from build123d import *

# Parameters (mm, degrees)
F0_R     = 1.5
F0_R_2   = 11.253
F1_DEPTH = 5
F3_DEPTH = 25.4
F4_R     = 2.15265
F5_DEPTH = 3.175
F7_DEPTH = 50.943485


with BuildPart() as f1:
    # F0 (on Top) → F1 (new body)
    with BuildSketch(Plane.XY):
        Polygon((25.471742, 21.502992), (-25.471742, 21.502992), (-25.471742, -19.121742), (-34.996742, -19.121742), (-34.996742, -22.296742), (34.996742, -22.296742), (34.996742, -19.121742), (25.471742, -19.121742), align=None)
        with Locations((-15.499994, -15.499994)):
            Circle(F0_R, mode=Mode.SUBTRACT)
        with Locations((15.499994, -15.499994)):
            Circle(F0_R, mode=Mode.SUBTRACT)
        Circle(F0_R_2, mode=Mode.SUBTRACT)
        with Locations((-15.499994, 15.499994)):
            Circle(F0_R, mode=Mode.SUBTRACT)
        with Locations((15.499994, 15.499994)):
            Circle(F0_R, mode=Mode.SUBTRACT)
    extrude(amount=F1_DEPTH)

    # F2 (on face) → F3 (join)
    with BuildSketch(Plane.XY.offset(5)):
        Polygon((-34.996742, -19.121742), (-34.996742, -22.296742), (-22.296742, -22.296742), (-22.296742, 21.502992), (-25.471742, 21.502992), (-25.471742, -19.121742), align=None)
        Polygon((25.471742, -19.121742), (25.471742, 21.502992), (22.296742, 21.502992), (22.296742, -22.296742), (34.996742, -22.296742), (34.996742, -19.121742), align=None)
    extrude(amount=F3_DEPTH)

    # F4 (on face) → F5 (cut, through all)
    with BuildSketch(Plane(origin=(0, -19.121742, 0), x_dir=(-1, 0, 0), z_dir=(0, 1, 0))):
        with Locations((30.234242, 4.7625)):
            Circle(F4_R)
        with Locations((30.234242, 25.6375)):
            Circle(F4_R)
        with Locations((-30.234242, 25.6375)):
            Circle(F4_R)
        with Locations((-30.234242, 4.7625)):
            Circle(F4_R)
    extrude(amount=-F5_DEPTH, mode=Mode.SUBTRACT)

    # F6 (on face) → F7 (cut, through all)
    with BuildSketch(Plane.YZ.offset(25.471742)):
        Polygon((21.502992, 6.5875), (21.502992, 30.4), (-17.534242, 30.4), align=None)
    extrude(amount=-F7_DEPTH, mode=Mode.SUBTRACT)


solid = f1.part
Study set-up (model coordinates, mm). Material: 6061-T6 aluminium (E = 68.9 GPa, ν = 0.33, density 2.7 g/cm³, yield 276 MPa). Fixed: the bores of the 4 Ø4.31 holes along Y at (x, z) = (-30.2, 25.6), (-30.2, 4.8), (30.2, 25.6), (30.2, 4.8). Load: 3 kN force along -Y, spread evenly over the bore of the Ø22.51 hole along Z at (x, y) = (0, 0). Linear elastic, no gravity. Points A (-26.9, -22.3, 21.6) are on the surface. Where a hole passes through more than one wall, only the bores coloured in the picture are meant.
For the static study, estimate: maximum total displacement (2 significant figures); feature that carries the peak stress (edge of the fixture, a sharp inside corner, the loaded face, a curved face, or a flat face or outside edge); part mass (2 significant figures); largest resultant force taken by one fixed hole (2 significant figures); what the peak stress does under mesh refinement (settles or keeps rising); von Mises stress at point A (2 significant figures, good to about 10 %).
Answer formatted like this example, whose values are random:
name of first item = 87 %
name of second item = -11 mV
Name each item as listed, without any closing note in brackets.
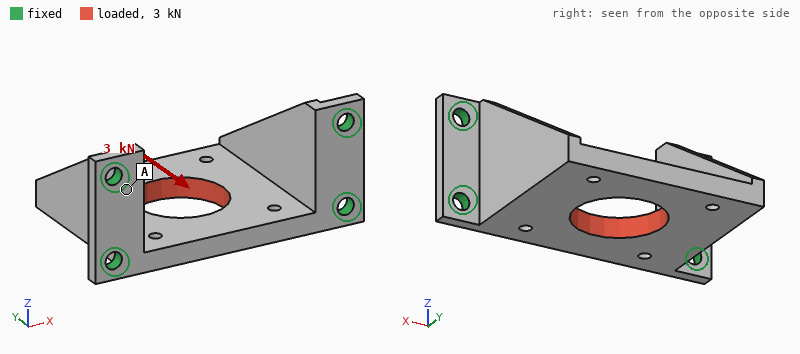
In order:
maximum total displacement = 81 µm
feature that carries the peak stress = edge of the fixture
part mass = 40 g
largest resultant force taken by one fixed hole = 1.8 kN
what the peak stress does under mesh refinement = keeps rising
von Mises stress at point A = 21 MPa
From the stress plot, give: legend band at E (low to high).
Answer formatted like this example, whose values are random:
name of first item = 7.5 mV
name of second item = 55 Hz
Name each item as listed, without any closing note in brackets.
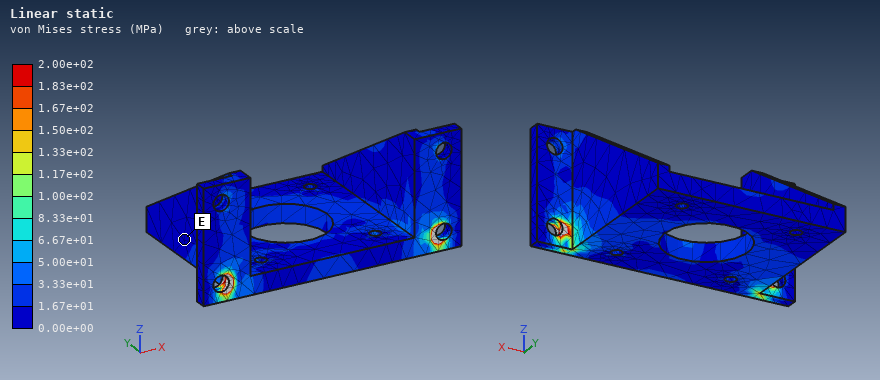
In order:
legend band at E = 0.00e+00 to 1.67e+01 MPa
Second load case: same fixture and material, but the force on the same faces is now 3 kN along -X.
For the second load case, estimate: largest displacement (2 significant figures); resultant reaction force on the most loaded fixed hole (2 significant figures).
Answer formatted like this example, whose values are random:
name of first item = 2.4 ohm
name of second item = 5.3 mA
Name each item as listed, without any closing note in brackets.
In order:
largest displacement = 71 µm
resultant reaction force on the most loaded fixed hole = 1.9 kN
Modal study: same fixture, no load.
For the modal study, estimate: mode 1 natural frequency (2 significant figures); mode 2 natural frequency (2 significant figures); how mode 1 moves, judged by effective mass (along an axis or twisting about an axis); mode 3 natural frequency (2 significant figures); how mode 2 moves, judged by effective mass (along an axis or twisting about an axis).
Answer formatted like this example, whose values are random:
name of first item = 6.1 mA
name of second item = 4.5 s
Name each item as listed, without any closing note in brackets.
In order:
mode 1 natural frequency = 4100 Hz
mode 2 natural frequency = 5800 Hz
how mode 1 moves, judged by effective mass = along Z
mode 3 natural frequency = 8000 Hz
how mode 2 moves, judged by effective mass = along X
